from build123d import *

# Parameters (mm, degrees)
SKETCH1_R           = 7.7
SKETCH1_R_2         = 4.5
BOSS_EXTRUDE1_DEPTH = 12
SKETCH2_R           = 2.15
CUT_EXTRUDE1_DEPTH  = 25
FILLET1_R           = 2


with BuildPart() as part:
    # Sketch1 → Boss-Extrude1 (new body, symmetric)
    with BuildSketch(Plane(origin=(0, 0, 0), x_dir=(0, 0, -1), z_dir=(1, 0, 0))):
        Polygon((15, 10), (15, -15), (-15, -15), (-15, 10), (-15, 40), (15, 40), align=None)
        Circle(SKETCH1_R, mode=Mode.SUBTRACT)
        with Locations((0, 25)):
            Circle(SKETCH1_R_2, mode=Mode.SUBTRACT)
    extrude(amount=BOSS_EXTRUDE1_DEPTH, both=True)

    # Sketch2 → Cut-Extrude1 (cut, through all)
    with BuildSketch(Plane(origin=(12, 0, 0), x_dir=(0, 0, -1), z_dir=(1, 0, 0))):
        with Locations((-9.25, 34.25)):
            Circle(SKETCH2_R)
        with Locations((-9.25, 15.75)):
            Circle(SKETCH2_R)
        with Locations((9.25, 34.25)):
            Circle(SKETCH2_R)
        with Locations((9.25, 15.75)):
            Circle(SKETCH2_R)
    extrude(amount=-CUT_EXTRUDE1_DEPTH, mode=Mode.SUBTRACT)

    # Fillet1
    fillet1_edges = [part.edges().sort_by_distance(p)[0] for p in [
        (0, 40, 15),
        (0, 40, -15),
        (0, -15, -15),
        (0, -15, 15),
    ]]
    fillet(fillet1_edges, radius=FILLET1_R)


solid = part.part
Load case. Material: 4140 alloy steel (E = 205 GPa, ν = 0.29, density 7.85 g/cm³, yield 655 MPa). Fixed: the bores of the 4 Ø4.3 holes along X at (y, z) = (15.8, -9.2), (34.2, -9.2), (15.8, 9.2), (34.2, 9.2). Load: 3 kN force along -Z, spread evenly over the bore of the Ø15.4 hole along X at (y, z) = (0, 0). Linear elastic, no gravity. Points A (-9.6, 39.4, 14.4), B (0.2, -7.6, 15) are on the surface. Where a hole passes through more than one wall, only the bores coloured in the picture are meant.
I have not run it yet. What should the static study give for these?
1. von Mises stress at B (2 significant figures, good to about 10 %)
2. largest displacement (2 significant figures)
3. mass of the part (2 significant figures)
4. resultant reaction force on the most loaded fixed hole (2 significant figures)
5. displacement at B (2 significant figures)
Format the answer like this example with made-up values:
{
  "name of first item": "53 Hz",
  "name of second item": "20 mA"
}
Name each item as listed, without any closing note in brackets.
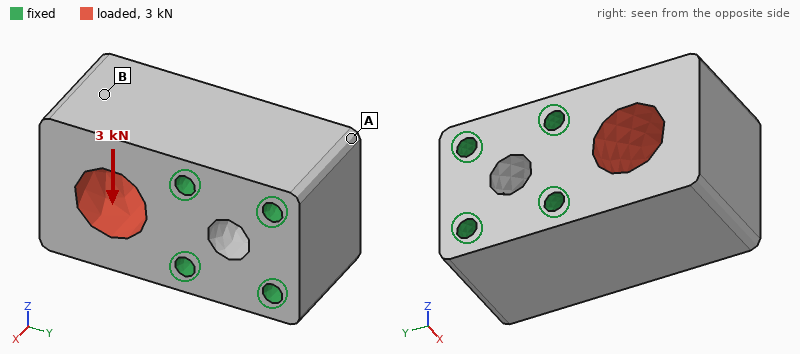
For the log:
{
  "von Mises stress at B": "6.7 MPa",
  "largest displacement": "4.4 µm",
  "mass of the part": "250 g",
  "resultant reaction force on the most loaded fixed hole": "2.3 kN",
  "displacement at B": "3.8 µm"
}
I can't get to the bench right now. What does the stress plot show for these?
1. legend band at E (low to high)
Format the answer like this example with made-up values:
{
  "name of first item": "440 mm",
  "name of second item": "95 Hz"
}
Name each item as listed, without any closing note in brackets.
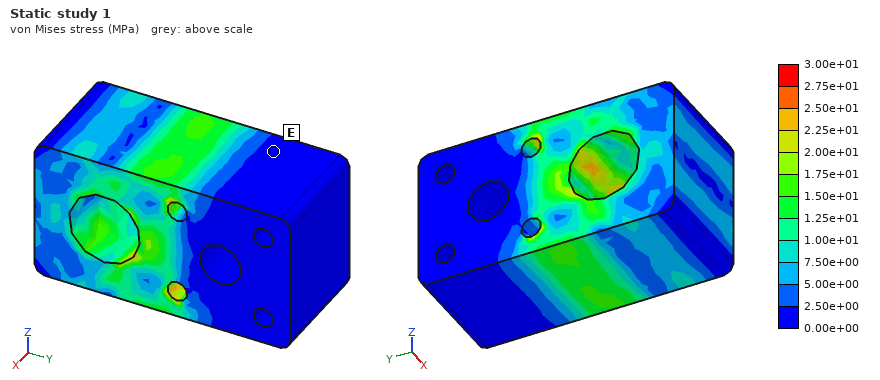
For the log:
{
  "legend band at E": "0.00e+00 to 2.50e+00 MPa"
}
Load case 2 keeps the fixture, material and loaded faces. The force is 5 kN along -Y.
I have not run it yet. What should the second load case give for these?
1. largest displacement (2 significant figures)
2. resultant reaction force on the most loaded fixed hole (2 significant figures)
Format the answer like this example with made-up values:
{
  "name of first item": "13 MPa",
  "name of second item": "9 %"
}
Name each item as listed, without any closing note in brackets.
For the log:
{
  "largest displacement": "1.6 µm",
  "resultant reaction force on the most loaded fixed hole": "2.4 kN"
}
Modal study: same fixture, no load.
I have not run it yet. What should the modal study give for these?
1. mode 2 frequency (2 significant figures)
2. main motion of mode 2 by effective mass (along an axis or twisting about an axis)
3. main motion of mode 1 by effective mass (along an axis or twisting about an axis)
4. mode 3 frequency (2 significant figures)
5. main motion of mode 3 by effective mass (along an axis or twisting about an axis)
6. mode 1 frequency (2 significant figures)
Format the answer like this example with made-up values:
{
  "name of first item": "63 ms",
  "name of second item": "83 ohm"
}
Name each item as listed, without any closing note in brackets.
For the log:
{
  "mode 2 frequency": "14 kHz",
  "main motion of mode 2 by effective mass": "along X",
  "main motion of mode 1 by effective mass": "along Z",
  "mode 3 frequency": "20 kHz",
  "main motion of mode 3 by effective mass": "twisting about Y",
  "mode 1 frequency": "13 kHz"
}
